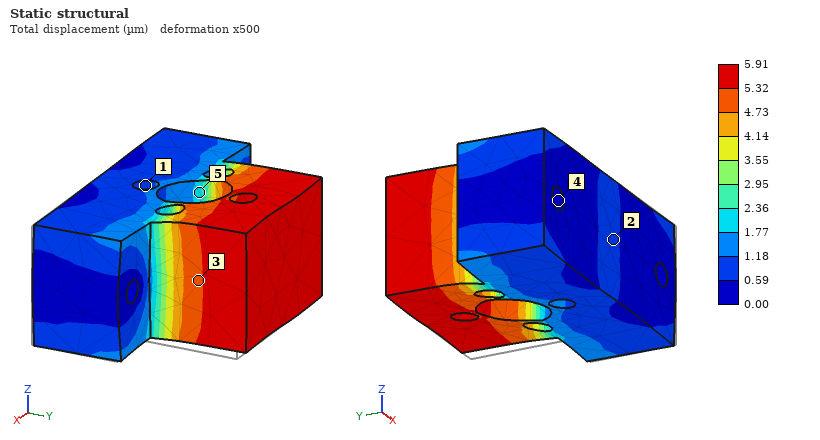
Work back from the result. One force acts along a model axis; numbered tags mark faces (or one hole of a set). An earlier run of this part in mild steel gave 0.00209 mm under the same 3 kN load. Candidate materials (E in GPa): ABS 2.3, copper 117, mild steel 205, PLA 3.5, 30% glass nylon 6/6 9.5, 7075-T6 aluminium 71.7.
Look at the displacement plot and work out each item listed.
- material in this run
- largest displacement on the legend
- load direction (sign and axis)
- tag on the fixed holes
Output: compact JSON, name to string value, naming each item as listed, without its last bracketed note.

{"material in this run": "7075-T6 aluminium", "largest displacement on the legend": "5.91 µm", "load direction": "-X", "tag on the fixed holes": "4"}
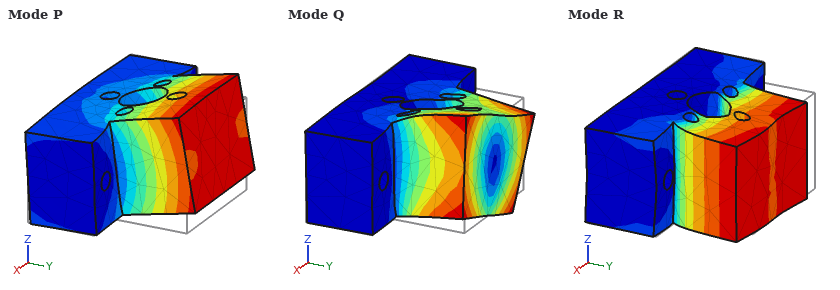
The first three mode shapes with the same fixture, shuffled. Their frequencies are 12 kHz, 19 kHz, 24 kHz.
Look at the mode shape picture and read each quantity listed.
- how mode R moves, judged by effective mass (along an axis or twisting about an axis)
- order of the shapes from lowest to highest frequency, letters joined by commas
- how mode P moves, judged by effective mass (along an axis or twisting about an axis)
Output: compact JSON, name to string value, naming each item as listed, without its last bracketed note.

{"how mode R moves, judged by effective mass": "along X", "order of the shapes from lowest to highest frequency, letters joined by commas": "P, R, Q", "how mode P moves, judged by effective mass": "along Z"}
